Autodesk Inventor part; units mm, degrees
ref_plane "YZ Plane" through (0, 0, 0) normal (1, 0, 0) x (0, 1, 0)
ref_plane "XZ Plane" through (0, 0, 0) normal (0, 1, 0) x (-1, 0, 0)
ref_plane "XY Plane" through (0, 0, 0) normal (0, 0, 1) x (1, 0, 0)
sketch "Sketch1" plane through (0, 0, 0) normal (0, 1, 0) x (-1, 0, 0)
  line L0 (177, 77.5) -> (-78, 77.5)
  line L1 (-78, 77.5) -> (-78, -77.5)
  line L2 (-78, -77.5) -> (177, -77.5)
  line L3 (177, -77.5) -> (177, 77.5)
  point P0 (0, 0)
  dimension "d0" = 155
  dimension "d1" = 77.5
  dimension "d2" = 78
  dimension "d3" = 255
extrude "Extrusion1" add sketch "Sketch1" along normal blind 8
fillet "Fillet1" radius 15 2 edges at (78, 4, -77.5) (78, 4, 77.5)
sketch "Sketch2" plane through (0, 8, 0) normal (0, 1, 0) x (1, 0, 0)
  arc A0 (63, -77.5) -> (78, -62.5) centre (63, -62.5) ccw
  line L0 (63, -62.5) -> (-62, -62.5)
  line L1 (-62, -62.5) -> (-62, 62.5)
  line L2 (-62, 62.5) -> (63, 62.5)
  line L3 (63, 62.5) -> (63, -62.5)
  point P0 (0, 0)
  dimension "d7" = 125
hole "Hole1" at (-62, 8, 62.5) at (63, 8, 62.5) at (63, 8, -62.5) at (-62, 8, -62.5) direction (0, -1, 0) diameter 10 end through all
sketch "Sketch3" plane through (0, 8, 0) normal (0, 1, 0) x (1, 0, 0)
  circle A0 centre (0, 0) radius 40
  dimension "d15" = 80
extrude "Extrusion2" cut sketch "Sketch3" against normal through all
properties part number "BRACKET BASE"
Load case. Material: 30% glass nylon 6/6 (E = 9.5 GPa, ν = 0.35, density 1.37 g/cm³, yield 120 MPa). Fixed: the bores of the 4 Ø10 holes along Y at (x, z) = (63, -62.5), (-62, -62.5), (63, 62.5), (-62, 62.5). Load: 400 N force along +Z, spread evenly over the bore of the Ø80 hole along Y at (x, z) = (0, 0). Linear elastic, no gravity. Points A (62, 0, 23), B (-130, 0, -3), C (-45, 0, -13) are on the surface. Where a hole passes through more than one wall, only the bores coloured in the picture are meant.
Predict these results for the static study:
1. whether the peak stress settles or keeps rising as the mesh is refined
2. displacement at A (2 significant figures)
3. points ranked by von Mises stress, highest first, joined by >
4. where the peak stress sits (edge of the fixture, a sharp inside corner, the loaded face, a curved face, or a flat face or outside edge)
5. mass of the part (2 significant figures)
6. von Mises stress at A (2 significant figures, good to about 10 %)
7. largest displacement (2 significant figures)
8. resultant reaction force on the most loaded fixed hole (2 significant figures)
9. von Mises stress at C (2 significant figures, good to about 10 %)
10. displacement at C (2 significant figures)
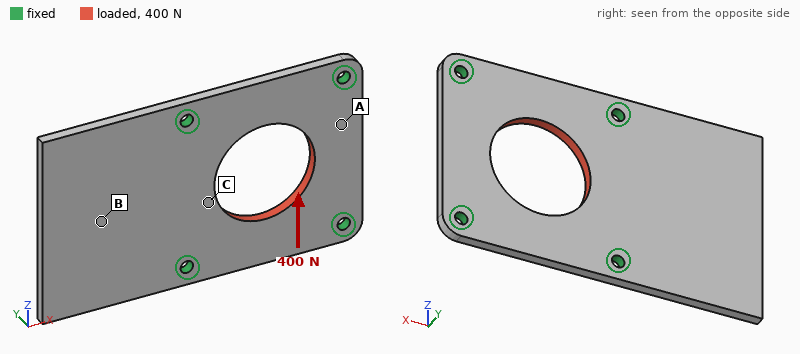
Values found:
keeps rising
1.2 µm
C > A > B
edge of the fixture
370 g
0.23 MPa
3.9 µm
110 N
0.36 MPa
1.8 µm
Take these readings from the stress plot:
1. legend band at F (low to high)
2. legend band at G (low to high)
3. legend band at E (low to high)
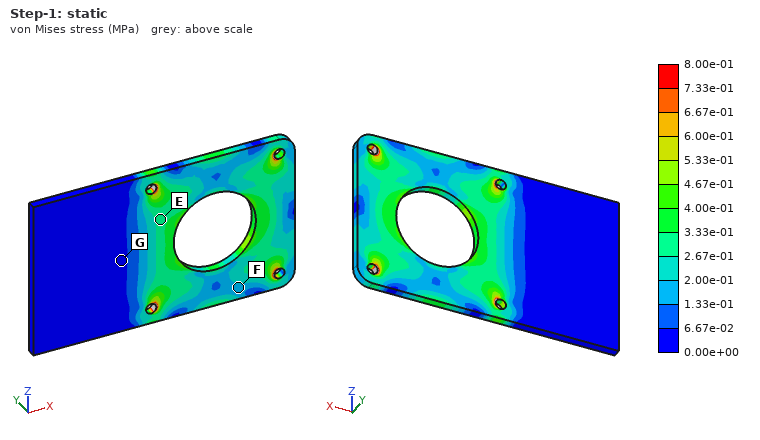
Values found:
1.33e-01 to 2.00e-01 MPa
0.00e+00 to 6.67e-02 MPa
2.67e-01 to 3.33e-01 MPa
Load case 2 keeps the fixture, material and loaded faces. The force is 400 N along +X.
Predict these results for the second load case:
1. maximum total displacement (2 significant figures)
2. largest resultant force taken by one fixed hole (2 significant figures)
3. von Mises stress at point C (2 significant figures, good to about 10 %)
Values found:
4.4 µm
110 N
0.17 MPa
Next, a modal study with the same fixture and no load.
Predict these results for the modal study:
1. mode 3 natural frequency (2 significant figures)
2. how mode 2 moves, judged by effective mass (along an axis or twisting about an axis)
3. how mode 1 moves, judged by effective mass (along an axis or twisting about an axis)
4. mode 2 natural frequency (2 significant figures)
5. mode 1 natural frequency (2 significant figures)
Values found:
1100 Hz
twisting about X
along Y
510 Hz
230 Hz
